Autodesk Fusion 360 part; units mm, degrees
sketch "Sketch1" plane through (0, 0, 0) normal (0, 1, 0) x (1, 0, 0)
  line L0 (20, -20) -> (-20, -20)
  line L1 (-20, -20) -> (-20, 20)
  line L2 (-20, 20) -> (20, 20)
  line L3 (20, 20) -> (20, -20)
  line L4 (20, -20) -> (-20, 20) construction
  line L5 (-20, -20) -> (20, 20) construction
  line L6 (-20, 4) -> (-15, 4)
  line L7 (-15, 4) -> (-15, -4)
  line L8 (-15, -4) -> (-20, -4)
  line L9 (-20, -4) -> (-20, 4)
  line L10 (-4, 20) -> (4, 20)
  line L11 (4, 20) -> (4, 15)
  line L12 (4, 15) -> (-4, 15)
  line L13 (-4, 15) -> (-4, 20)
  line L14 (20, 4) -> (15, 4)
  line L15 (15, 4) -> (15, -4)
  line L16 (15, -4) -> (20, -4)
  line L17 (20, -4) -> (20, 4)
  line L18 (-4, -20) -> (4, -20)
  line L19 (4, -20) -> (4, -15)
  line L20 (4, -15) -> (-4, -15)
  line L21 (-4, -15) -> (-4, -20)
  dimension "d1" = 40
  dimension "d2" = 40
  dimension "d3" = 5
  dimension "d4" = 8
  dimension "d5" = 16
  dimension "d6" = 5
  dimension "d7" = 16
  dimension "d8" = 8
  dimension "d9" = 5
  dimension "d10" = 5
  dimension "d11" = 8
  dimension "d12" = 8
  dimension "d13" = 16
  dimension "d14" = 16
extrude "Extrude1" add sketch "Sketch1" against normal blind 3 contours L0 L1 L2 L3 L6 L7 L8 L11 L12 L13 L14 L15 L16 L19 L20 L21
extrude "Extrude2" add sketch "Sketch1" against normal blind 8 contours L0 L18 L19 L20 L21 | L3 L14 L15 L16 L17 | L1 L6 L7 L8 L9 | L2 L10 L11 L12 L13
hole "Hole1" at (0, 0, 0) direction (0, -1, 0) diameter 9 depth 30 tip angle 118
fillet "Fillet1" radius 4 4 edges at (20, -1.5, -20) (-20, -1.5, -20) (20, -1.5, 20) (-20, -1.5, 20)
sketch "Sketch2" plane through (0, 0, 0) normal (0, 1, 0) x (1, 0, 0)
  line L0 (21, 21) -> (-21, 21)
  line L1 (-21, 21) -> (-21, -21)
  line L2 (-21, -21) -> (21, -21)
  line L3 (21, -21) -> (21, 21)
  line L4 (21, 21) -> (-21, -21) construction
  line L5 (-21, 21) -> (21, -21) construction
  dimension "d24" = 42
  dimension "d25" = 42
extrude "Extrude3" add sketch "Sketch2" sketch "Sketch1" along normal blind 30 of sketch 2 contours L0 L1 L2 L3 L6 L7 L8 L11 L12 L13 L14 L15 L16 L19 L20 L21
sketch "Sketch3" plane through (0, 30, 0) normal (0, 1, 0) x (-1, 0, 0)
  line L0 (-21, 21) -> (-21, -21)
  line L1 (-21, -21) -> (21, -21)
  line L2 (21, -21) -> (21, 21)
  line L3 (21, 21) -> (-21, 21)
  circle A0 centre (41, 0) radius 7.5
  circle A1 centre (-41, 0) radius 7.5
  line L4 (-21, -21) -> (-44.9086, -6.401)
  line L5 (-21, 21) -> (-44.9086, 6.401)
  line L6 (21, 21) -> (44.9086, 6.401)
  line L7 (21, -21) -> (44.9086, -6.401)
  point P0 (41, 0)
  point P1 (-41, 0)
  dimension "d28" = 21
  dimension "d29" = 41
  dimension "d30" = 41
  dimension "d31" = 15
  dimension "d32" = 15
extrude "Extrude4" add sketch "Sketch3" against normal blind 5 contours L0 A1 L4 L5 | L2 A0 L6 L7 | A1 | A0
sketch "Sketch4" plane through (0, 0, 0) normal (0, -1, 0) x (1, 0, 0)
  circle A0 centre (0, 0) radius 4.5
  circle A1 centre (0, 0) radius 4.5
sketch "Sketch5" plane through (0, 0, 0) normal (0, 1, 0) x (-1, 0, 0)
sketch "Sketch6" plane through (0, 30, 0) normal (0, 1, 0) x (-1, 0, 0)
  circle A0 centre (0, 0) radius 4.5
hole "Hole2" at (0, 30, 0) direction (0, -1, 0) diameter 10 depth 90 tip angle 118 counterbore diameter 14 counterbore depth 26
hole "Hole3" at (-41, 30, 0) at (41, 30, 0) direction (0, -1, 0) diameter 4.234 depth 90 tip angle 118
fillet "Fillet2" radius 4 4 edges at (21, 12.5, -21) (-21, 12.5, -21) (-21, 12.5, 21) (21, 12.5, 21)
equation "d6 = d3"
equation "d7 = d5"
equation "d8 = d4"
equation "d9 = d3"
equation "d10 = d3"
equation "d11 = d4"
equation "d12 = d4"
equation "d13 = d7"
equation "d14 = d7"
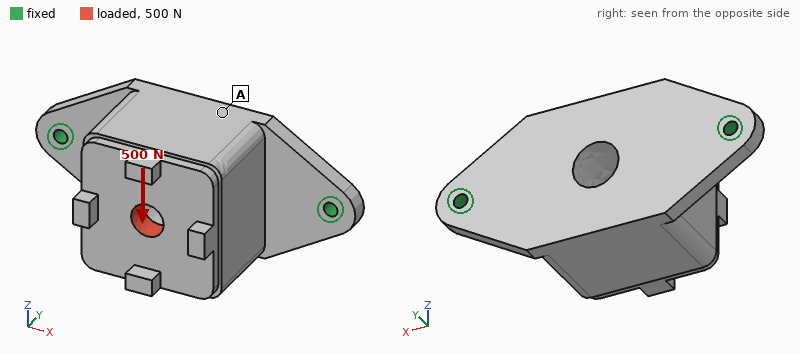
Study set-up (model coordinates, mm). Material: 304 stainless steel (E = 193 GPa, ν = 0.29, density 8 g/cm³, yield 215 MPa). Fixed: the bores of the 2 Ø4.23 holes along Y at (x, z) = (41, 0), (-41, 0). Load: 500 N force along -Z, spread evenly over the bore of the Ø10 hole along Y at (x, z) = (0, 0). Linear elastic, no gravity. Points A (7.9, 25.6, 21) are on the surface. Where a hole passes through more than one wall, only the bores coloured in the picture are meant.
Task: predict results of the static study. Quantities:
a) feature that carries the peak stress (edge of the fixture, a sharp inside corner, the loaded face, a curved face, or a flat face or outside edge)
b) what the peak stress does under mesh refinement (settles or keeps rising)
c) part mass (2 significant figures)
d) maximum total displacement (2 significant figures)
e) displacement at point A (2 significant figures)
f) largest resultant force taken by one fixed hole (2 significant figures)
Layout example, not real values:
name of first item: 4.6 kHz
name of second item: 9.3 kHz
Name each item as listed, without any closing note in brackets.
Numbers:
feature that carries the peak stress: edge of the fixture
what the peak stress does under mesh refinement: keeps rising
part mass: 480 g
maximum total displacement: 67 µm
displacement at point A: 34 µm
largest resultant force taken by one fixed hole: 250 N
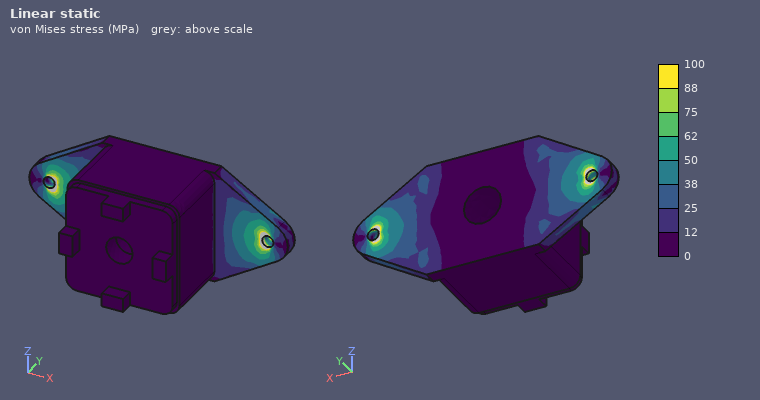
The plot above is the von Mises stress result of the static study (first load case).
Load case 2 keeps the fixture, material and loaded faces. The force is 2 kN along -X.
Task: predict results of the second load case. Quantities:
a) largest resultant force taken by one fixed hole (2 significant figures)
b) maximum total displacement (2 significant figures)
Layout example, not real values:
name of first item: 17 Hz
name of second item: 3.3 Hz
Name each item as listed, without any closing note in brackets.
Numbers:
largest resultant force taken by one fixed hole: 1.3 kN
maximum total displacement: 24 µm
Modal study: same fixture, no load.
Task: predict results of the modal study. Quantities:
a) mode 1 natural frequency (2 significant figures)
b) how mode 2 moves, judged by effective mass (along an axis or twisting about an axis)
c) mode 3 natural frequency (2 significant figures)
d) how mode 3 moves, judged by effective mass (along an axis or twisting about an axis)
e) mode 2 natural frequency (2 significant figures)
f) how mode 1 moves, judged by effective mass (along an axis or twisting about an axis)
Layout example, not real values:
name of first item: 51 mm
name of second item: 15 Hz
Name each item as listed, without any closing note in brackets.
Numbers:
mode 1 natural frequency: 1000 Hz
how mode 2 moves, judged by effective mass: along Y
mode 3 natural frequency: 3400 Hz
how mode 3 moves, judged by effective mass: along X
mode 2 natural frequency: 2300 Hz
how mode 1 moves, judged by effective mass: along Z
